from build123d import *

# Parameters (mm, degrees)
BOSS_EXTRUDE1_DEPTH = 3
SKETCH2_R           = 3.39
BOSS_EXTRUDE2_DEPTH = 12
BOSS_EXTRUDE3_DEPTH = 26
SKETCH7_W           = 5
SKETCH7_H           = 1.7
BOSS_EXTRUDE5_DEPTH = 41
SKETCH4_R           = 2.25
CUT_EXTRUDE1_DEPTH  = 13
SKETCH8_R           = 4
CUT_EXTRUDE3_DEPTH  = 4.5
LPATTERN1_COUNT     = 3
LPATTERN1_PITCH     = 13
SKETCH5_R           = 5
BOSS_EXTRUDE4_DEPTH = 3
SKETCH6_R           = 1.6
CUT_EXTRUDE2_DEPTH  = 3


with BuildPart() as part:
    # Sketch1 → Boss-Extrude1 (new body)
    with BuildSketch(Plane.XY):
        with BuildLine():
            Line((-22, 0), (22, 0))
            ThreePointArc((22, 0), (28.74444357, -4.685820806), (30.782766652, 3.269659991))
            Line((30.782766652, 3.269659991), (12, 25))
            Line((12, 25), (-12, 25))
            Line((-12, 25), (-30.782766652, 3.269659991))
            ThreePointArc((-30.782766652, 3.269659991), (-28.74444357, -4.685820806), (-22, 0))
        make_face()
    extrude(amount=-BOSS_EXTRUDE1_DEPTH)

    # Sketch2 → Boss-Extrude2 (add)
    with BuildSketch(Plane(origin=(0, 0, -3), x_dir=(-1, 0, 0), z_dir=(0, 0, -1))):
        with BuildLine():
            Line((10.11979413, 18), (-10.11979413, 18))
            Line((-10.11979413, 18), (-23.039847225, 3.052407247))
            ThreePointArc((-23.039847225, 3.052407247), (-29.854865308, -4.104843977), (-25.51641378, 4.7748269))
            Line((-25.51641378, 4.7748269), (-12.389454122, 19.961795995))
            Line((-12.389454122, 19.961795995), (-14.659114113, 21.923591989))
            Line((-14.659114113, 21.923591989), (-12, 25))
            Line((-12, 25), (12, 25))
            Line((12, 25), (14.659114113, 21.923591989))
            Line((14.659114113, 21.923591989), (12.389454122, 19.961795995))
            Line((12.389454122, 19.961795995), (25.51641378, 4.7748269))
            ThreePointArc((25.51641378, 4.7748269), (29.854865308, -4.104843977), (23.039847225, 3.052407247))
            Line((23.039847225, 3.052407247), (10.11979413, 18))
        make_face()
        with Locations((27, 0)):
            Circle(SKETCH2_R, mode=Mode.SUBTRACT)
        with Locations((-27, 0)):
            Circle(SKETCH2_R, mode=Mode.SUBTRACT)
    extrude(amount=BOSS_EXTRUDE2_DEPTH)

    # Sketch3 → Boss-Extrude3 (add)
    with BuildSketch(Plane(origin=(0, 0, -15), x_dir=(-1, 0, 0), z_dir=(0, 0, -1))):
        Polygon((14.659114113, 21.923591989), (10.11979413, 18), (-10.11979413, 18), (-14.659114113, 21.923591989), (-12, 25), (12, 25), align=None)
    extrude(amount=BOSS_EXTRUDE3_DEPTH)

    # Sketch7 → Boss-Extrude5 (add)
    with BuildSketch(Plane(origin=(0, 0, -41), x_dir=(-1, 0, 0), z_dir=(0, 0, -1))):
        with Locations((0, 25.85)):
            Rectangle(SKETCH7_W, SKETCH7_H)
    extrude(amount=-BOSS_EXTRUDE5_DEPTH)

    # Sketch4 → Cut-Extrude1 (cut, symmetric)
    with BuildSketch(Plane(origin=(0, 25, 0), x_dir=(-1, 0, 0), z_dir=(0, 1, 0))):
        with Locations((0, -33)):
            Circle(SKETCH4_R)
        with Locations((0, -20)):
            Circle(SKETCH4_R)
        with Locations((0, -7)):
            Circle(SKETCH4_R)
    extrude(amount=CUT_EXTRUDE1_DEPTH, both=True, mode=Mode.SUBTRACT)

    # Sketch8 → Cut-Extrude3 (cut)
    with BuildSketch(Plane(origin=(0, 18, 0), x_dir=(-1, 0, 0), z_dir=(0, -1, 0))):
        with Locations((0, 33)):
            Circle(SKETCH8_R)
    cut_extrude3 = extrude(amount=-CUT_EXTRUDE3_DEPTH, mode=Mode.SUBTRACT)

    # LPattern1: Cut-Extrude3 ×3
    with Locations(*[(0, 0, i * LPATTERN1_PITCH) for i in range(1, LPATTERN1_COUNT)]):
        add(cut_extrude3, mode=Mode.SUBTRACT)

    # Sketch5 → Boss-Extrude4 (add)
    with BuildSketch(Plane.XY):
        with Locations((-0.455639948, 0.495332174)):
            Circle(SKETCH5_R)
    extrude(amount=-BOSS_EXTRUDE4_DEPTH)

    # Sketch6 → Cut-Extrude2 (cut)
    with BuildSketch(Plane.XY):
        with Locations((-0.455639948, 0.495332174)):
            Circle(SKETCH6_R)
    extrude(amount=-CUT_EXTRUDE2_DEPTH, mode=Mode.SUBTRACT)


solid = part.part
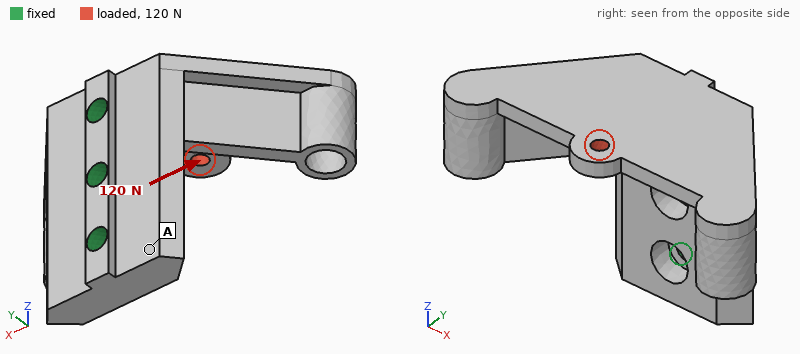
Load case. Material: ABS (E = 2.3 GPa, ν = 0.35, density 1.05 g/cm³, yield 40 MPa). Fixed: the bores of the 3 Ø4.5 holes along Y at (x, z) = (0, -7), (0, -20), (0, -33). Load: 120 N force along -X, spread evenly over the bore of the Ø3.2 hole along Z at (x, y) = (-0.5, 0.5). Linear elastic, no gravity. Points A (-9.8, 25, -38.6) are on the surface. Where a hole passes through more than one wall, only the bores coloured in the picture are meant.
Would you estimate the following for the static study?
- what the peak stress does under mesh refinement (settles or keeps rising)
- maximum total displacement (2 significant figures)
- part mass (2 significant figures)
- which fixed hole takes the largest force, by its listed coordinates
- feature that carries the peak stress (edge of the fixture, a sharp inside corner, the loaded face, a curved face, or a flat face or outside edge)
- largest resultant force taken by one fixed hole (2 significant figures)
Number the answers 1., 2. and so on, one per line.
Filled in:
1. keeps rising
2. 0.96 mm
3. 13 g
4. (0, -7)
5. edge of the fixture
6. 110 N
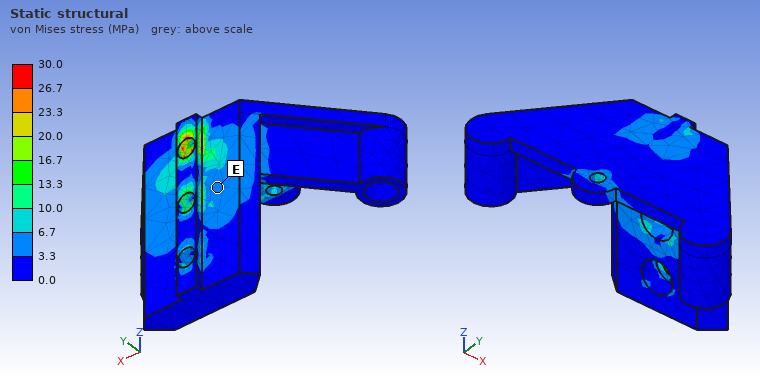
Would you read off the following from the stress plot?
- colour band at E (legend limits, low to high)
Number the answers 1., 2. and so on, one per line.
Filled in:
1. 3.3 to 6.7 MPa
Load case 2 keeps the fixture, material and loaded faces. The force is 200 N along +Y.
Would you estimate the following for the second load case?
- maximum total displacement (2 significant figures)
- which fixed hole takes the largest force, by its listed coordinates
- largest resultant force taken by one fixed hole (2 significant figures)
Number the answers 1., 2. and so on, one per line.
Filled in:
1. 0.14 mm
2. (0, -7)
3. 230 N
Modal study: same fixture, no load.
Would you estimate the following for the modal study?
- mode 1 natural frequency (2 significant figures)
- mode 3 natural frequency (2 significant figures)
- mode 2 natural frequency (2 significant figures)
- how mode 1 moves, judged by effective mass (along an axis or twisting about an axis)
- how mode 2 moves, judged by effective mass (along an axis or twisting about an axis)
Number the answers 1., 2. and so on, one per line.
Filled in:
1. 860 Hz
2. 2000 Hz
3. 1700 Hz
4. along X
5. along Z
